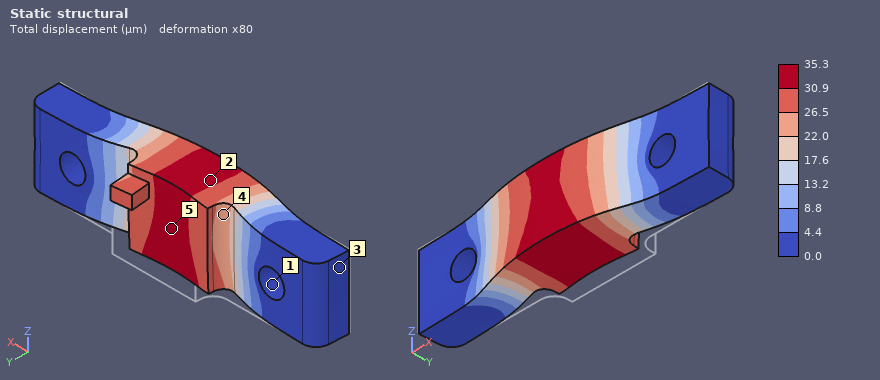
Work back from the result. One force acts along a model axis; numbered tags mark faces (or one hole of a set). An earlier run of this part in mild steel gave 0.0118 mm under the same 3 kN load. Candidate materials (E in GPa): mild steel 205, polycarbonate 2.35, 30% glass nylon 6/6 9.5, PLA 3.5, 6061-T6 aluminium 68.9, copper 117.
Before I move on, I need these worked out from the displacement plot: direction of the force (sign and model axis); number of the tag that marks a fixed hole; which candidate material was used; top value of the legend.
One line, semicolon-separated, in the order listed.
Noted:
-Y; 1; 6061-T6 aluminium; 35.3 µm
